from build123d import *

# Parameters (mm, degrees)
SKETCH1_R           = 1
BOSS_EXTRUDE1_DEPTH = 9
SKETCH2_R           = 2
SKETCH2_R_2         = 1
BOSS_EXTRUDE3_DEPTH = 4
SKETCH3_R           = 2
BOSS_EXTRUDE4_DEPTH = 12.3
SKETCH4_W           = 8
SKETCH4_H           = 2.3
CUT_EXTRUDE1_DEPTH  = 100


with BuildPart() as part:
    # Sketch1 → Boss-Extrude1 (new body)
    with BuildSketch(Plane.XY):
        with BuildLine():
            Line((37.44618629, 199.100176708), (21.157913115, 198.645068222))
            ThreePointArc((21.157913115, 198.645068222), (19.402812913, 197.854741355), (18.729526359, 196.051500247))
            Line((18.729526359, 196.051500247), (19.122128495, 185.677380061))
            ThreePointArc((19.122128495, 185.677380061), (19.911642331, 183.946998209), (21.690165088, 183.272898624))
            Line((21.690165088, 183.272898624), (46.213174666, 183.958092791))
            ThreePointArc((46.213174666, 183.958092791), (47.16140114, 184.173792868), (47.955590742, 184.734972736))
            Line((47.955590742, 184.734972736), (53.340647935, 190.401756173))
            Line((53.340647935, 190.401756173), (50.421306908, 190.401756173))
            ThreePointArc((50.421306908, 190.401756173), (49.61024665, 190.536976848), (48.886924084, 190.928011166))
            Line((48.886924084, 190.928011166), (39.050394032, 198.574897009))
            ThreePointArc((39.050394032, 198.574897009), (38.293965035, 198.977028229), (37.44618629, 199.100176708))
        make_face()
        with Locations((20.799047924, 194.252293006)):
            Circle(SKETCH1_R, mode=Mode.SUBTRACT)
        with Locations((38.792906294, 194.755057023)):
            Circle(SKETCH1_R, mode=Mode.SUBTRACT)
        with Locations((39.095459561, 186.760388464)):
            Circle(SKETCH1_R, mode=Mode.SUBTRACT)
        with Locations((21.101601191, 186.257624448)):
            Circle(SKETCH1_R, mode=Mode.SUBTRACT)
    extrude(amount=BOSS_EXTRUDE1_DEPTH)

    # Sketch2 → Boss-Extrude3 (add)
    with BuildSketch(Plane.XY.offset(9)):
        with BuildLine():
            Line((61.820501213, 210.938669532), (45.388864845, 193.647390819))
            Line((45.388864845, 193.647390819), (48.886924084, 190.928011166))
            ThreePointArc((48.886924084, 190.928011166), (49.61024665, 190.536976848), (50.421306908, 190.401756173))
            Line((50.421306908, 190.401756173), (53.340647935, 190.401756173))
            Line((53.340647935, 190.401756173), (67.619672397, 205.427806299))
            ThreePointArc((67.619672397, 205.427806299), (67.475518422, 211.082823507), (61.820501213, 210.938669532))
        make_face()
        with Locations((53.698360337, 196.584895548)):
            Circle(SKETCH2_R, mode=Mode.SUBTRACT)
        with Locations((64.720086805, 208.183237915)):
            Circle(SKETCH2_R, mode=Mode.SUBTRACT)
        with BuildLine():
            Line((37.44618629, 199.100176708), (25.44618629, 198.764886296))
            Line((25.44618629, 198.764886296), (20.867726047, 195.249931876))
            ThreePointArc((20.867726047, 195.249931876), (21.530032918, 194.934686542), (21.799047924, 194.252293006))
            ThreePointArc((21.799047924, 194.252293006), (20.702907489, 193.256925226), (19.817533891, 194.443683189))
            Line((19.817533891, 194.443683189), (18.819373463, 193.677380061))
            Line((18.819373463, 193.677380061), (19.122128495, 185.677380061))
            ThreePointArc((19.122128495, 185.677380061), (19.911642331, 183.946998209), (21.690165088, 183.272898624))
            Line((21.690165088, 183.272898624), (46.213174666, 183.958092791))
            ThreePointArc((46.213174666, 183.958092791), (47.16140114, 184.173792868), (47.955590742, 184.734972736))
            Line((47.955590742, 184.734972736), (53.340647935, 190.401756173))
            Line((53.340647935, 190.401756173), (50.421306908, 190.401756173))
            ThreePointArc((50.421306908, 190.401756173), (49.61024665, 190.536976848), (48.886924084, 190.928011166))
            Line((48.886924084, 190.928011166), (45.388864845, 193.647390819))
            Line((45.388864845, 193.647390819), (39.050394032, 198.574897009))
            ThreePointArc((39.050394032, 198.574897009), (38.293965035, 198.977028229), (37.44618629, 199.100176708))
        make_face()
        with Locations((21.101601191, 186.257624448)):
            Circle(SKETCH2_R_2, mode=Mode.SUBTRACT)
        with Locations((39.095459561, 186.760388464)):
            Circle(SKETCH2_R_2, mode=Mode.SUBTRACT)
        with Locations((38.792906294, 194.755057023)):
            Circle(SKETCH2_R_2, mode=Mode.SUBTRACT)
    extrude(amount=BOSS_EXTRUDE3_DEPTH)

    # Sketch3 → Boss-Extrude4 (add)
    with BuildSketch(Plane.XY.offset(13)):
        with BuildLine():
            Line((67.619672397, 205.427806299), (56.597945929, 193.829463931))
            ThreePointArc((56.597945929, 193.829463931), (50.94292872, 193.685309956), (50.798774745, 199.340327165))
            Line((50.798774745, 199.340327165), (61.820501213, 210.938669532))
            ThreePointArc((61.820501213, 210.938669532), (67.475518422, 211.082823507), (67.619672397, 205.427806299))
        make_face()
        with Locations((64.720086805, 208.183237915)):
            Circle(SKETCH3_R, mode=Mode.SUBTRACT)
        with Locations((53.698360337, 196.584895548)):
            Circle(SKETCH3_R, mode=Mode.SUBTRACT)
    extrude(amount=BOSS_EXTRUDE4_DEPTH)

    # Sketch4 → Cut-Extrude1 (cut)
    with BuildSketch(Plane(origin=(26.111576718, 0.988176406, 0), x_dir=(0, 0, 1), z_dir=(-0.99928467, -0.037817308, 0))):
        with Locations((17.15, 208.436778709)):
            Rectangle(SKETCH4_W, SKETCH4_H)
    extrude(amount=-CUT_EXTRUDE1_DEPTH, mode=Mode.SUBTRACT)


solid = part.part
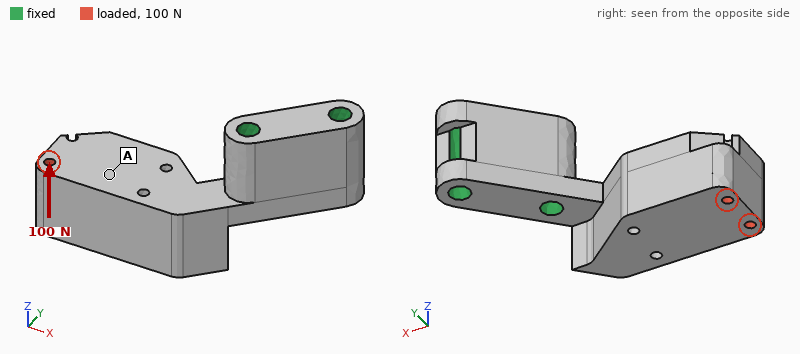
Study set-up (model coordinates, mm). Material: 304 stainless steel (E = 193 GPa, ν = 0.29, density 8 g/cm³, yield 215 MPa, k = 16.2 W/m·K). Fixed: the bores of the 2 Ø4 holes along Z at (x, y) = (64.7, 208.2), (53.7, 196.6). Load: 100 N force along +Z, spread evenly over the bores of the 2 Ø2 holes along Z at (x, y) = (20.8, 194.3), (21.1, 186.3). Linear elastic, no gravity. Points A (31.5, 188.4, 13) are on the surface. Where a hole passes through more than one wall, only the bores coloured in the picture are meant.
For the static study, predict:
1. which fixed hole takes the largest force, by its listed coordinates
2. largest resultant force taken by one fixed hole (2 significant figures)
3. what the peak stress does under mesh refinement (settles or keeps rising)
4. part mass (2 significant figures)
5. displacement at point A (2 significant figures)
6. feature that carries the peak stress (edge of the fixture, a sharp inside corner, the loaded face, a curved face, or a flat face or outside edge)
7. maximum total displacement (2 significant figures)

(53.7, 196.6)
110 N
keeps rising
62 g
39 µm
a sharp inside corner
68 µm
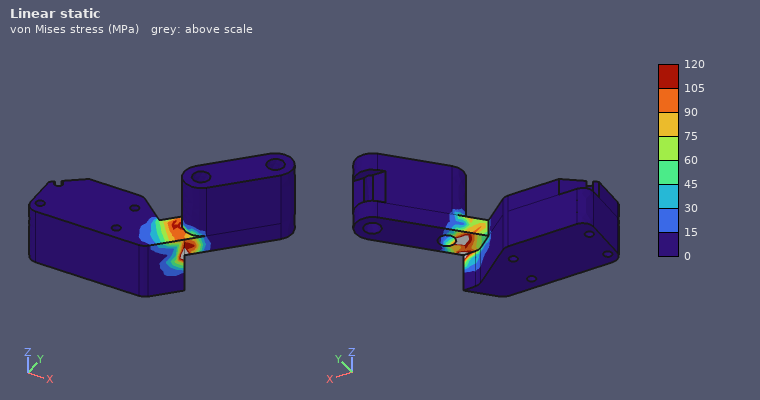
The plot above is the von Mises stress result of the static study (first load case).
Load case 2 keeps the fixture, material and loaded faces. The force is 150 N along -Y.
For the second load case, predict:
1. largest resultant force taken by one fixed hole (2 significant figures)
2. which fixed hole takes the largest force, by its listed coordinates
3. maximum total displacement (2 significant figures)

190 N
(53.7, 196.6)
53 µm
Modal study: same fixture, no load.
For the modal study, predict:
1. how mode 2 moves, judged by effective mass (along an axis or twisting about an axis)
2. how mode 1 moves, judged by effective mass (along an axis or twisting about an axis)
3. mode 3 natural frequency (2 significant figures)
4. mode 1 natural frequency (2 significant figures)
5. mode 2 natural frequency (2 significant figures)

along Y
along Z
4800 Hz
1500 Hz
2200 Hz
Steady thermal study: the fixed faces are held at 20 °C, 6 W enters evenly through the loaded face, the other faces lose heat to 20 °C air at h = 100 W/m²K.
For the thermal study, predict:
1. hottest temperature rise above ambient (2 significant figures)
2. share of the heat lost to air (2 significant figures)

44 K
86 %
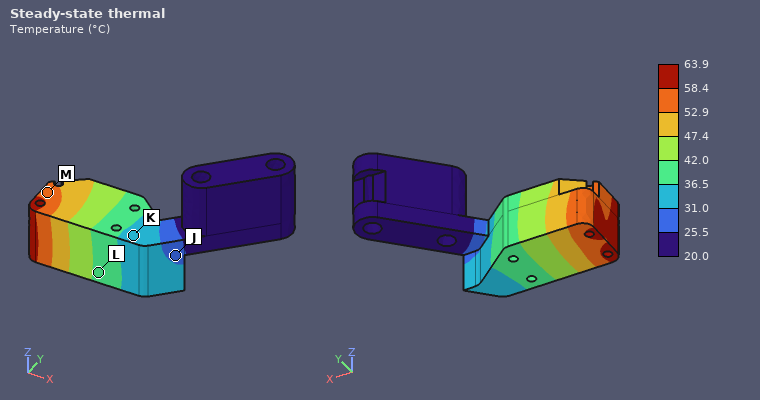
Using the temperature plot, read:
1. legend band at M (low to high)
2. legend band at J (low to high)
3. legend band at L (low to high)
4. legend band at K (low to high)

52.9 to 58.4 °C
25.5 to 31.0 °C
36.5 to 42.0 °C
31.0 to 36.5 °C
